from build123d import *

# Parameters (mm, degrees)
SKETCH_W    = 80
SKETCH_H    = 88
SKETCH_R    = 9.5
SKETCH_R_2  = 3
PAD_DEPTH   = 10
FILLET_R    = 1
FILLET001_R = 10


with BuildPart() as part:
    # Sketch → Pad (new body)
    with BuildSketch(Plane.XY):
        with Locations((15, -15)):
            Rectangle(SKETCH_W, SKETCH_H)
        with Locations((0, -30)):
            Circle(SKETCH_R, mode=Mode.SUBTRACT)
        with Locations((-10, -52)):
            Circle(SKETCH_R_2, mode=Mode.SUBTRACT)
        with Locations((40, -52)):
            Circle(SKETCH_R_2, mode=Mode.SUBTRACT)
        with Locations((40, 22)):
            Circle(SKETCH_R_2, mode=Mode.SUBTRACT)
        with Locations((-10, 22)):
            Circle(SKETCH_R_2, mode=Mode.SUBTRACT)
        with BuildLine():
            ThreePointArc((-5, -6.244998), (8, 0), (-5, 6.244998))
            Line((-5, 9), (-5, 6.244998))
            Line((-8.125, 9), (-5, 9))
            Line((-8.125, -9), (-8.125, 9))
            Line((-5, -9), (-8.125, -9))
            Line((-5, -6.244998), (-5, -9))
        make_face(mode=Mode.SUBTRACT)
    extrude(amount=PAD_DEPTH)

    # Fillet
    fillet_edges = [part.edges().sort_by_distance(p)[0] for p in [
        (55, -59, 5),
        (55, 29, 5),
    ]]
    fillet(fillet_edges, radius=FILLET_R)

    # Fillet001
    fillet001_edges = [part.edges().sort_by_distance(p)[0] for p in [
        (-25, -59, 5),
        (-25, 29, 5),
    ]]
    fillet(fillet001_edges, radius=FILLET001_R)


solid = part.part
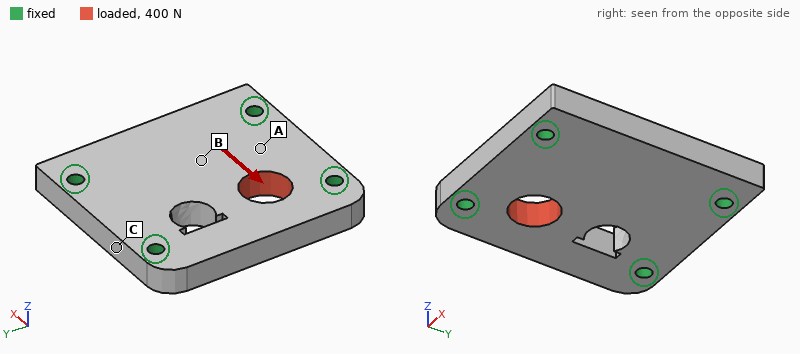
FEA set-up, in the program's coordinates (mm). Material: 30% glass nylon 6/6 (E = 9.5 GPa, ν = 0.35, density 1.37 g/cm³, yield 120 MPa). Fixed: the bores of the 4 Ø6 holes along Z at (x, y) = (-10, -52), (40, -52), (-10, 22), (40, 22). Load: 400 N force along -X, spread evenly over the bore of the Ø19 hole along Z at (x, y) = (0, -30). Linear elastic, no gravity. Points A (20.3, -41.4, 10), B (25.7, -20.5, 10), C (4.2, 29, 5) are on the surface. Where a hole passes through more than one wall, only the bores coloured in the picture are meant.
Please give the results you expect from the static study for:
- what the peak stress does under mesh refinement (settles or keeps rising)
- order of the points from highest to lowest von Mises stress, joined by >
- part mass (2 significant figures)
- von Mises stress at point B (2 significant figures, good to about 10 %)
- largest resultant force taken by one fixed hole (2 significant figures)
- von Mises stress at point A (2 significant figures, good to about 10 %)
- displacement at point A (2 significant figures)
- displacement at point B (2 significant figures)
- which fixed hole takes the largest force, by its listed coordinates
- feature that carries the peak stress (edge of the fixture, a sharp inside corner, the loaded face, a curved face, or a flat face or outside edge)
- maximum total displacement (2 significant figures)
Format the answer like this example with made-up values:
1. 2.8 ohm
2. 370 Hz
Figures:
1. keeps rising
2. A > B > C
3. 87 g
4. 0.35 MPa
5. 160 N
6. 0.65 MPa
7. 1.5 µm
8. 2.5 µm
9. (-10, -52)
10. edge of the fixture
11. 5.0 µm
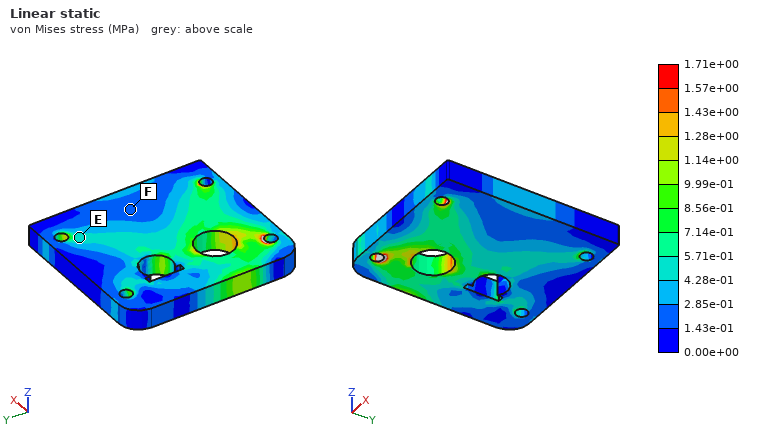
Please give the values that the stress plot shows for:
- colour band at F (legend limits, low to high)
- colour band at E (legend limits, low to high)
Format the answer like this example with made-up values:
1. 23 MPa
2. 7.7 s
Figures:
1. 1.43e-01 to 2.85e-01 MPa
2. 4.28e-01 to 5.71e-01 MPa
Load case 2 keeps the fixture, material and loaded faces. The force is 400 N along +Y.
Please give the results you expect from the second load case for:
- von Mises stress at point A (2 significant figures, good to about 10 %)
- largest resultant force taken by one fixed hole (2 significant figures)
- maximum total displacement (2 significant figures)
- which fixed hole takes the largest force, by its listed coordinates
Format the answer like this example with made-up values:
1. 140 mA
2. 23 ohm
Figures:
1. 0.47 MPa
2. 190 N
3. 3.3 µm
4. (-10, -52)
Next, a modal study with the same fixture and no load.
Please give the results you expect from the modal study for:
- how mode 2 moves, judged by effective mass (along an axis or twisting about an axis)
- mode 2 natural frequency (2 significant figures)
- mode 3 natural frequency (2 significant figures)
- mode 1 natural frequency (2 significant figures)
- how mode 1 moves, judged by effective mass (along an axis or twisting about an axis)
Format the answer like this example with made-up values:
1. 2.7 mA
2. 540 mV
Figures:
1. twisting about Y
2. 4600 Hz
3. 6100 Hz
4. 3800 Hz
5. along Z
